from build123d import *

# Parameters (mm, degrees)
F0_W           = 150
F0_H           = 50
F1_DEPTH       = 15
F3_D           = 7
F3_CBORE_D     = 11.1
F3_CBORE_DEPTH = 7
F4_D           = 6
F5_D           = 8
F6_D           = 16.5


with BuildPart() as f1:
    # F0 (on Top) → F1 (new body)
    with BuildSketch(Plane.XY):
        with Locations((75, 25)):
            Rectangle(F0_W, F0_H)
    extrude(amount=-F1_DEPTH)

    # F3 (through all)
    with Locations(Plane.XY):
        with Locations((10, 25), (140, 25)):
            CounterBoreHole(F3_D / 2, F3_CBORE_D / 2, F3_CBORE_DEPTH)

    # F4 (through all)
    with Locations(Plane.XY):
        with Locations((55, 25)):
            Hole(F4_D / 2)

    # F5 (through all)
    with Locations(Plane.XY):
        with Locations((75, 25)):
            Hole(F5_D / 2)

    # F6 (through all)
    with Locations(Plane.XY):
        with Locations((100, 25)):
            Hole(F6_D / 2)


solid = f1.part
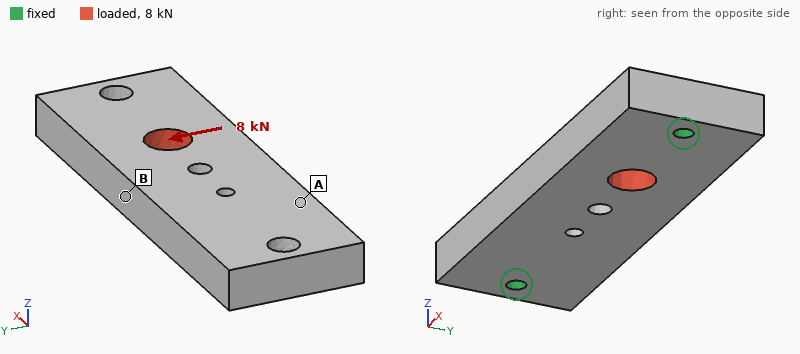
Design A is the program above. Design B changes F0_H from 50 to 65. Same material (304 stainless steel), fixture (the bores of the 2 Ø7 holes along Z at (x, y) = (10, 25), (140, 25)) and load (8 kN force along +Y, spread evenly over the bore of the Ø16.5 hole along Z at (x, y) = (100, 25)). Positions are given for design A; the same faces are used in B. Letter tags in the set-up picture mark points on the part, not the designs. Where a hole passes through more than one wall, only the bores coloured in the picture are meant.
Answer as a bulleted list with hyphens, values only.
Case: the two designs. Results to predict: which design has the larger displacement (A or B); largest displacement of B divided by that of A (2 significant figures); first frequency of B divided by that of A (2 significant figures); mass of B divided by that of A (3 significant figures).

- A
- 0.74
- 0.91
- 1.32
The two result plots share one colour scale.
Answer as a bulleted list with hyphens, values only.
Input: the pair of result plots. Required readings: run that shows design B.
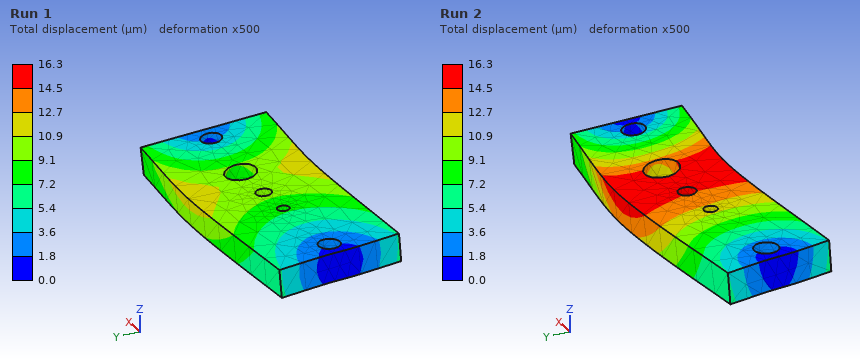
- Run 1
